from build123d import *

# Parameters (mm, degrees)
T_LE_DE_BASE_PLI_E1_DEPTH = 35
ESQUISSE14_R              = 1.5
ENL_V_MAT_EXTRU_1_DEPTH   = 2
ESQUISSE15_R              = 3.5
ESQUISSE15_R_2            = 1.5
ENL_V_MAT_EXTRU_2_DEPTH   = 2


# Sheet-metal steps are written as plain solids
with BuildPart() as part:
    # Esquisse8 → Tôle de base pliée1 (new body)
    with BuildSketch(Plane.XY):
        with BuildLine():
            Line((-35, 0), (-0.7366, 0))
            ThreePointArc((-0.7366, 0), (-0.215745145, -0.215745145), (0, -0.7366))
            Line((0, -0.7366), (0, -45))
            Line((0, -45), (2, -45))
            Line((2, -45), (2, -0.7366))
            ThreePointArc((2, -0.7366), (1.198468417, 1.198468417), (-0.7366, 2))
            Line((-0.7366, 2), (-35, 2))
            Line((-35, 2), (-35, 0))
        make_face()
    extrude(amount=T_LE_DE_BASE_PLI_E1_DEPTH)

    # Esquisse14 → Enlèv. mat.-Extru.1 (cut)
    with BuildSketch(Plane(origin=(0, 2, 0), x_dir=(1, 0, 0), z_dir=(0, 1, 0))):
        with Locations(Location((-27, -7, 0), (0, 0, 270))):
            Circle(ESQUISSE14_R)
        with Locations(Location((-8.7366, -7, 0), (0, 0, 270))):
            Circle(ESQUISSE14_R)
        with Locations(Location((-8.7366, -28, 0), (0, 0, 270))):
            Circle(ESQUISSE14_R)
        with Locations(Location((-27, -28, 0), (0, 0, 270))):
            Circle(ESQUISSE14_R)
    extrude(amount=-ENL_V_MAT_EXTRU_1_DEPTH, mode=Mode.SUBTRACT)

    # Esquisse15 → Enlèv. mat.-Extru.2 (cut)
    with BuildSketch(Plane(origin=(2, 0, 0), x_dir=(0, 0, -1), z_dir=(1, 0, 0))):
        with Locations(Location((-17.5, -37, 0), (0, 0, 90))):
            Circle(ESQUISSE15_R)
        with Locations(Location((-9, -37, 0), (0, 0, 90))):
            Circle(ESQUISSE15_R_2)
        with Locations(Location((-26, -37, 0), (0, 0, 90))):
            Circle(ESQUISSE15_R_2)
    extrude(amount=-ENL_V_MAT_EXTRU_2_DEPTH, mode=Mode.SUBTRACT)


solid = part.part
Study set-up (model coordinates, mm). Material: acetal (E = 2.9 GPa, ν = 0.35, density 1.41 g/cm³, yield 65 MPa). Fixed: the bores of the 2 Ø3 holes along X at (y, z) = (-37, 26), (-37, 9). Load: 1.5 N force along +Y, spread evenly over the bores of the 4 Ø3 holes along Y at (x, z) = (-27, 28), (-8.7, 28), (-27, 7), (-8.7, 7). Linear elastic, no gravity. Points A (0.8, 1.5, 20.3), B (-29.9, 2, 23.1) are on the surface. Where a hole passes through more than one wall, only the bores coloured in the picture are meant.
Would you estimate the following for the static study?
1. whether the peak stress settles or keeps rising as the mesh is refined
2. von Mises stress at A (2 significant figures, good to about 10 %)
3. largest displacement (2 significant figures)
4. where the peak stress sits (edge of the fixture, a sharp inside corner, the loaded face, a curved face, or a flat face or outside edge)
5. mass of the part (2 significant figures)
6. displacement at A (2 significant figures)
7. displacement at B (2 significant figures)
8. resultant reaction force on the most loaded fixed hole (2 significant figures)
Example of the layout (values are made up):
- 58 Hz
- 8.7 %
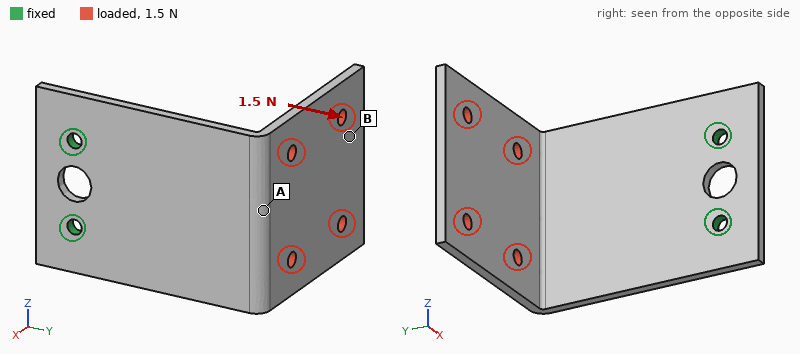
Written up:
- keeps rising
- 0.80 MPa
- 0.74 mm
- edge of the fixture
- 7.8 g
- 0.30 mm
- 0.65 mm
- 0.76 N
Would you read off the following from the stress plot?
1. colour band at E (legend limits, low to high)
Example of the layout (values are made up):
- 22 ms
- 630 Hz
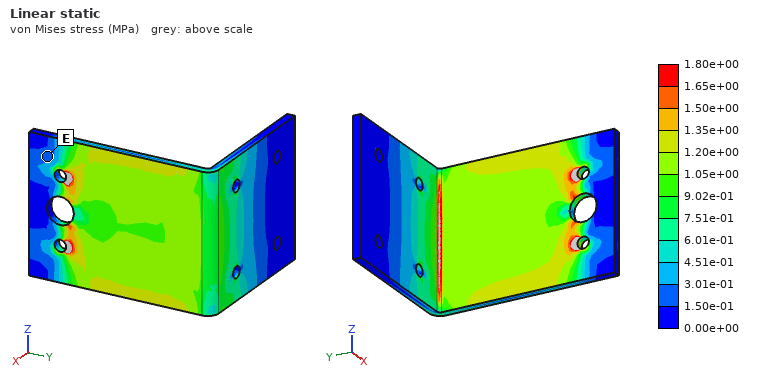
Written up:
- 1.50e-01 to 3.01e-01 MPa
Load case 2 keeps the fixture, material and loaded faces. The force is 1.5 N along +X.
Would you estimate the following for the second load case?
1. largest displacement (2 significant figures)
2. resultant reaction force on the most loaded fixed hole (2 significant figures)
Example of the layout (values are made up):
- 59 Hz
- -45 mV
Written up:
- 0.71 mm
- 0.75 N
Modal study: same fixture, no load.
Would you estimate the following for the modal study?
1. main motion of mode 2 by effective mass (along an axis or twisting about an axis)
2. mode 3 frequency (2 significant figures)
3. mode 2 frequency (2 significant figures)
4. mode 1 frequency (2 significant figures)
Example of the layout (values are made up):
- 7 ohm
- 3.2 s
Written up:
- along Z
- 330 Hz
- 220 Hz
- 120 Hz
